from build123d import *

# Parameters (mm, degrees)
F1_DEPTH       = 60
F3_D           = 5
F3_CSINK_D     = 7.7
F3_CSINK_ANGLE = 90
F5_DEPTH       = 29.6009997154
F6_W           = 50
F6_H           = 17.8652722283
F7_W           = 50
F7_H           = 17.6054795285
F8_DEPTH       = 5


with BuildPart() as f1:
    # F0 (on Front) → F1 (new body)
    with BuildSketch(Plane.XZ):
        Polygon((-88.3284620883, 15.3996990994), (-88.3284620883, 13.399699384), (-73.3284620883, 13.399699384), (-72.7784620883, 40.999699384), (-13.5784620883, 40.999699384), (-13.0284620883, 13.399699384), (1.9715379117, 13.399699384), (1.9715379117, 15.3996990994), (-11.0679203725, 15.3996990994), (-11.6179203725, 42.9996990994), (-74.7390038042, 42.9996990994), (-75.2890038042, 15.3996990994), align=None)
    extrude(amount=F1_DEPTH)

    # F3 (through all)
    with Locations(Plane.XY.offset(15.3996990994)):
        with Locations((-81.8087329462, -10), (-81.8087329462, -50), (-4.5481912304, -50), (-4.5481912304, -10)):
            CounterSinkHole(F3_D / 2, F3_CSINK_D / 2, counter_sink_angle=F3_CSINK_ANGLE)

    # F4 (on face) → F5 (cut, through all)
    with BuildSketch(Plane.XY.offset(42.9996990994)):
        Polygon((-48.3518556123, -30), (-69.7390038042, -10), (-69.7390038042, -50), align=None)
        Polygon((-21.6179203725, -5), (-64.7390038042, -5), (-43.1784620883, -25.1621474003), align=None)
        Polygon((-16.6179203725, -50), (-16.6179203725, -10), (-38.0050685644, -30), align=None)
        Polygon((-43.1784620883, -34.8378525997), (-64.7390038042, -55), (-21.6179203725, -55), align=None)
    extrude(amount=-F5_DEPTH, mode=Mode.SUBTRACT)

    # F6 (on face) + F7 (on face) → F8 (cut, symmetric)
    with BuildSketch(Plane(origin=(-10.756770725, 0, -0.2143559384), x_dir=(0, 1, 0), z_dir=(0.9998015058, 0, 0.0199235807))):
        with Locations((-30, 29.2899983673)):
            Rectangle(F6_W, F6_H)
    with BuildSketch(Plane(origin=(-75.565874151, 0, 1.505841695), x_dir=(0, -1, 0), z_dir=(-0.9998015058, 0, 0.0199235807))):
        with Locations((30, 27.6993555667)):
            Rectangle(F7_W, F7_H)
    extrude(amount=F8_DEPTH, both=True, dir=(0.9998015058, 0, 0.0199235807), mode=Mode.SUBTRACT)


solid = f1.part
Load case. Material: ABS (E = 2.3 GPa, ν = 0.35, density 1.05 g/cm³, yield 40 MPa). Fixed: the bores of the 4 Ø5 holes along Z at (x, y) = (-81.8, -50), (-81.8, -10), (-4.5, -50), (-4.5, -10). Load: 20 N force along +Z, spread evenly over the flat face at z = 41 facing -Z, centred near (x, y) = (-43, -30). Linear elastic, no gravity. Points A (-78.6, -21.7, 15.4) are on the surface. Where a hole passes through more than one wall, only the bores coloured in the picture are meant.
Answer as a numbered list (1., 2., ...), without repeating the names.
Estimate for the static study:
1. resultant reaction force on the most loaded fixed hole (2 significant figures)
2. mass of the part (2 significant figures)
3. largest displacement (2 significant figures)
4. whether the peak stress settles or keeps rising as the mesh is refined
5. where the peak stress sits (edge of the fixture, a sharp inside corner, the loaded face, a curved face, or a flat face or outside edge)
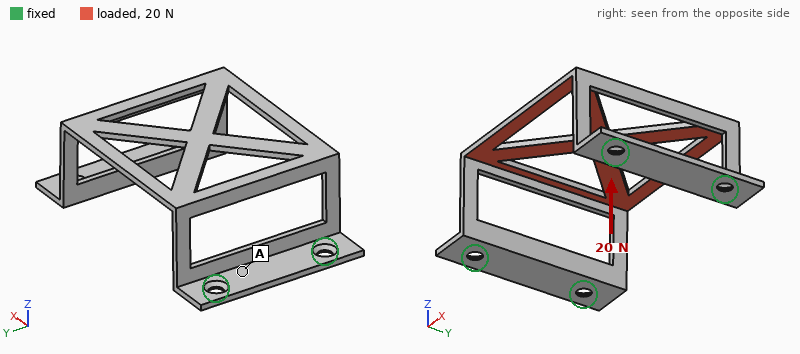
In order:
1. 7.1 N
2. 11 g
3. 0.98 mm
4. keeps rising
5. a sharp inside corner
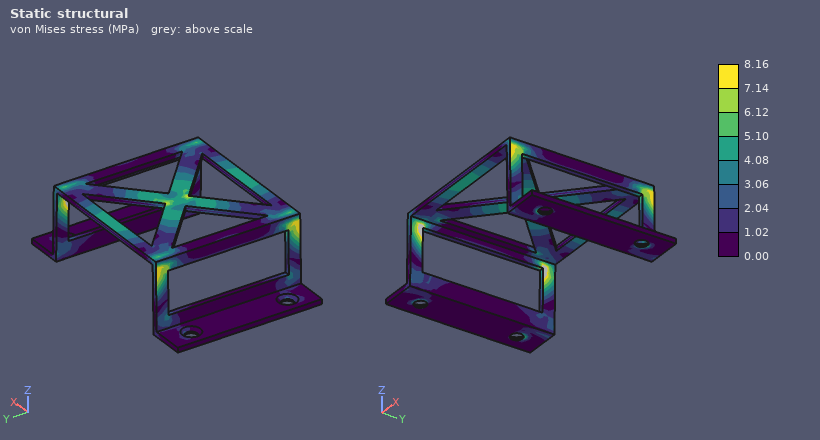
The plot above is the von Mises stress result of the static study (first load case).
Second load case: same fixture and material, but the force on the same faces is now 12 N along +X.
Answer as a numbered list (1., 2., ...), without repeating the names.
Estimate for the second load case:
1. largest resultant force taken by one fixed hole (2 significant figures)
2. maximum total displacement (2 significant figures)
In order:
1. 3.6 N
2. 0.98 mm
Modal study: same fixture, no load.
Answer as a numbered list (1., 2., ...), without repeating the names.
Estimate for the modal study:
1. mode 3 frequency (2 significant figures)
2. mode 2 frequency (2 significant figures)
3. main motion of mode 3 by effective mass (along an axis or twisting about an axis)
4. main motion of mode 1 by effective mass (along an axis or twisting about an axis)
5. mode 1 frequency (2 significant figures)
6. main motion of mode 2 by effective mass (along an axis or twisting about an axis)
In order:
1. 560 Hz
2. 440 Hz
3. along Y
4. along X
5. 240 Hz
6. along Z
